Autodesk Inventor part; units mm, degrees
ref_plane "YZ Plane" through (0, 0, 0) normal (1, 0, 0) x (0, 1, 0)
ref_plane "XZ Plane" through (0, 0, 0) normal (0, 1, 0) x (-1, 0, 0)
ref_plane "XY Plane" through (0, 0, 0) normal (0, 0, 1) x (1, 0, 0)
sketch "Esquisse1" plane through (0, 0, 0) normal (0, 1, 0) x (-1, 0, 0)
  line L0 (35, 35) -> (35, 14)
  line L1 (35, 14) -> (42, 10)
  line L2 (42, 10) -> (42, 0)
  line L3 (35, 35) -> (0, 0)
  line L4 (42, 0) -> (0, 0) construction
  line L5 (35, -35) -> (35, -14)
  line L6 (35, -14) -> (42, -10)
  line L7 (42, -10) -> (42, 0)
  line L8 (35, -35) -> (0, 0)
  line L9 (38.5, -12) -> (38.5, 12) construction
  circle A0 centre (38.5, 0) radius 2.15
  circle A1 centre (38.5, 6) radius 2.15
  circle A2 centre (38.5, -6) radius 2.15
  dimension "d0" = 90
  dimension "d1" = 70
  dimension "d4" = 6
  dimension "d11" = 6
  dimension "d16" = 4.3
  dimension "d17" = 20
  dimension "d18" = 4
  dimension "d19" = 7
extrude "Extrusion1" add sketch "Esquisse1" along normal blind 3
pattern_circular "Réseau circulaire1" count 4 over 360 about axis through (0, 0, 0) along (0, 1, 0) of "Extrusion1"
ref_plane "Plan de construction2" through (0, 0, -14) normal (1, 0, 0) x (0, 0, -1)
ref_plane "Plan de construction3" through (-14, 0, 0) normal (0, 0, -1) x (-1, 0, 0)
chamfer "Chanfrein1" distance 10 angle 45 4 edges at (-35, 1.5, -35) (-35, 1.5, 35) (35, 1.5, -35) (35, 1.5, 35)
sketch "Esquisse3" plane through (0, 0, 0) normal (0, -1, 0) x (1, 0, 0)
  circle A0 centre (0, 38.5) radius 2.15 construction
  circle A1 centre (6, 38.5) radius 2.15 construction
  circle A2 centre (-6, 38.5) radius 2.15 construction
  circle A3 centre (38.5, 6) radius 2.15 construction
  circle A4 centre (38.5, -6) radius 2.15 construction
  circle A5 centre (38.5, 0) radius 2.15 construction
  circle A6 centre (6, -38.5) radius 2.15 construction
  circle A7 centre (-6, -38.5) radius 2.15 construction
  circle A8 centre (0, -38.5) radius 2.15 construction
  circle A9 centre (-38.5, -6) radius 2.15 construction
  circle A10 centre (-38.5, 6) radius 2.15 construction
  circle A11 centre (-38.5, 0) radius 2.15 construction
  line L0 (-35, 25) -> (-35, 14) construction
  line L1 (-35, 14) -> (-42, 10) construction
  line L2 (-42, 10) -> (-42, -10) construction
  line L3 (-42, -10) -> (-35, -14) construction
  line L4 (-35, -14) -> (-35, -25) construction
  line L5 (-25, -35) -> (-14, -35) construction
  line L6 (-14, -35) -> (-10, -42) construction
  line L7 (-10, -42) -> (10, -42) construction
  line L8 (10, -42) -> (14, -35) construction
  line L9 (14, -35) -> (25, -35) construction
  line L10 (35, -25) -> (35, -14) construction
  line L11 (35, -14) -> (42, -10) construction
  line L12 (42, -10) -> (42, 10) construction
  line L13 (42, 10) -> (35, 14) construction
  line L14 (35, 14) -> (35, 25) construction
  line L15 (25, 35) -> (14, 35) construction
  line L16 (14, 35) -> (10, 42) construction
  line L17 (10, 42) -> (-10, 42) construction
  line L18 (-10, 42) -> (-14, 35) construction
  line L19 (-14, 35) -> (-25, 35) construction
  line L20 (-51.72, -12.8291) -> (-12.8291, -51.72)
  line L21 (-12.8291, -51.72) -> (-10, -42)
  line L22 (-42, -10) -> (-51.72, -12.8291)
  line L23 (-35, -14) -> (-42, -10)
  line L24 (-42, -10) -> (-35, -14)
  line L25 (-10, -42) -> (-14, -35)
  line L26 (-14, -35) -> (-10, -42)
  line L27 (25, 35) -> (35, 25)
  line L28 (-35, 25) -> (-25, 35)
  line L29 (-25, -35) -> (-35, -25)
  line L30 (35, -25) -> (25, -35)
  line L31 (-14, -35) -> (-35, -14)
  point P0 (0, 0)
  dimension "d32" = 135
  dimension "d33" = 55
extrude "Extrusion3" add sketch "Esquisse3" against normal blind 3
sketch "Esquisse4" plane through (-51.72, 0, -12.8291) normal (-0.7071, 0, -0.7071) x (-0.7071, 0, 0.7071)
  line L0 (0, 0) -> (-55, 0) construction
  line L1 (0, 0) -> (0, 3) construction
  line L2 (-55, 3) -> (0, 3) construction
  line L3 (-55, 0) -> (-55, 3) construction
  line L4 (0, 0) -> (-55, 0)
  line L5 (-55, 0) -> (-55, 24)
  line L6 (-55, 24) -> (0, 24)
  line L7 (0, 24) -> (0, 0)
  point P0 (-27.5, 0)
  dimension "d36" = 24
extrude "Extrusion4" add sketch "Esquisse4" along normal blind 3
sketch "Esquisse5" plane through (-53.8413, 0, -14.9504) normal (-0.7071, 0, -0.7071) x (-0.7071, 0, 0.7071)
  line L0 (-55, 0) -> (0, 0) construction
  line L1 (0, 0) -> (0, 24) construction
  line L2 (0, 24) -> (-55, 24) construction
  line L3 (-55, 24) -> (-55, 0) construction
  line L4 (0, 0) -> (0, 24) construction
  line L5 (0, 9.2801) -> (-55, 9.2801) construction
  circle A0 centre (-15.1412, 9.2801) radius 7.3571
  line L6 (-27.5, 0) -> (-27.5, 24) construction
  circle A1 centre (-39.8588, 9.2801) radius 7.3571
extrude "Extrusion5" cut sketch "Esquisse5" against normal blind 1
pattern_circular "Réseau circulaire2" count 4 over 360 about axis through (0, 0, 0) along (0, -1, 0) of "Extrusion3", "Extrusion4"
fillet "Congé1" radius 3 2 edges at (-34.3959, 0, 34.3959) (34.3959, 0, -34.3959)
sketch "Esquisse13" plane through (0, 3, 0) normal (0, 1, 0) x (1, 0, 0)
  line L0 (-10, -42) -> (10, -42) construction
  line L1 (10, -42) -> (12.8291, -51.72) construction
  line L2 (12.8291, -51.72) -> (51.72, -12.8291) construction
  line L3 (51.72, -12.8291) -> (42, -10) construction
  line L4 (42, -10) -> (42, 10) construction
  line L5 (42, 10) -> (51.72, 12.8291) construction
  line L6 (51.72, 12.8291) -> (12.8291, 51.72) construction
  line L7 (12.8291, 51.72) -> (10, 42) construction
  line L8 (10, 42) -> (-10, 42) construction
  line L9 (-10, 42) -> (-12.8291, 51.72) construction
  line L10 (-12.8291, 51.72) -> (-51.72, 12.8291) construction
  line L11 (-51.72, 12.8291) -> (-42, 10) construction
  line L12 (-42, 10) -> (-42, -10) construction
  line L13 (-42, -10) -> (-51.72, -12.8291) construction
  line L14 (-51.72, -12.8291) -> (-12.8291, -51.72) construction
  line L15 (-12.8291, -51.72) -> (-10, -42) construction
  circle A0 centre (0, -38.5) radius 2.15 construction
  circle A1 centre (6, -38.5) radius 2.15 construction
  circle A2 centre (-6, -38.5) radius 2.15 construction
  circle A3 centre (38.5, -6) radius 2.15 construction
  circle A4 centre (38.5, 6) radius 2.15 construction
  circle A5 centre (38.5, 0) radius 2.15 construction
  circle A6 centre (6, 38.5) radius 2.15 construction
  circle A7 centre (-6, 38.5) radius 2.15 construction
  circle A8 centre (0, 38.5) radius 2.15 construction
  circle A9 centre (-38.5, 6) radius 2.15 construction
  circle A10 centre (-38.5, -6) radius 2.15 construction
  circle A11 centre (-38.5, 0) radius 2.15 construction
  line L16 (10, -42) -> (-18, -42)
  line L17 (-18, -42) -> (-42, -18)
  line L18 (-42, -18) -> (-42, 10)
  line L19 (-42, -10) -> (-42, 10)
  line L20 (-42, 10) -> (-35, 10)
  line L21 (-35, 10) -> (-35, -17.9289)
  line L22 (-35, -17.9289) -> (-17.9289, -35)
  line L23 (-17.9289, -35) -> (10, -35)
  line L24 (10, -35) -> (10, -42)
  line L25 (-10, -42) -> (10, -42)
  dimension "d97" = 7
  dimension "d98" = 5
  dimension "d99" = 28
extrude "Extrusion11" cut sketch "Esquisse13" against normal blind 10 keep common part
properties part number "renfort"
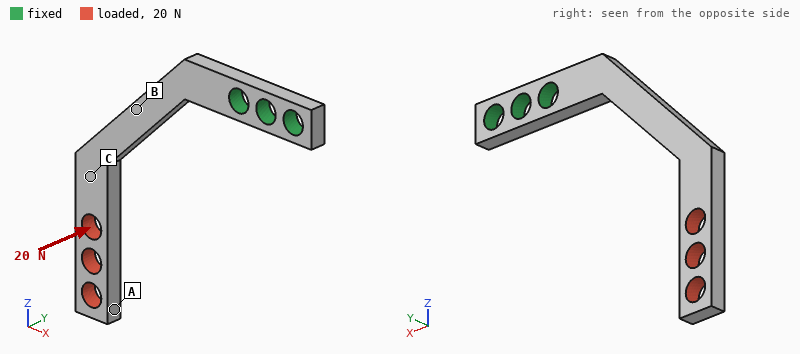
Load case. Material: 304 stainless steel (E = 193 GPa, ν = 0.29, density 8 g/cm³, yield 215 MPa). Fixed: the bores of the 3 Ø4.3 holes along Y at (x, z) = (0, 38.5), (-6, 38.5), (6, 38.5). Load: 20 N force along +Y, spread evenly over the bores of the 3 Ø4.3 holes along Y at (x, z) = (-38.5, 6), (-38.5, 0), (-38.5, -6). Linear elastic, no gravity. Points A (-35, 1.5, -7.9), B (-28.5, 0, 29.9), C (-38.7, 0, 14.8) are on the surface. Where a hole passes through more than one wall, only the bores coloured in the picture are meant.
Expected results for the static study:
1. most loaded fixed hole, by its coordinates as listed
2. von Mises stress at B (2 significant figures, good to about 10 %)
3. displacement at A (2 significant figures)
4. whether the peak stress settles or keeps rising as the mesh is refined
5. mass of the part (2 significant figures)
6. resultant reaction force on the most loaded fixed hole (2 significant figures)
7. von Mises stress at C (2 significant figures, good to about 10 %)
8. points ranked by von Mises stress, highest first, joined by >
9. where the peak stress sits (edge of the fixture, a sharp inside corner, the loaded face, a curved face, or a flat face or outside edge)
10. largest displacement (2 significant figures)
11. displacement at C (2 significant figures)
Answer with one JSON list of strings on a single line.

["(-6, 38.5)", "79 MPa", "0.47 mm", "keeps rising", "11 g", "22 N", "29 MPa", "B > C > A", "a sharp inside corner", "0.52 mm", "0.24 mm"]
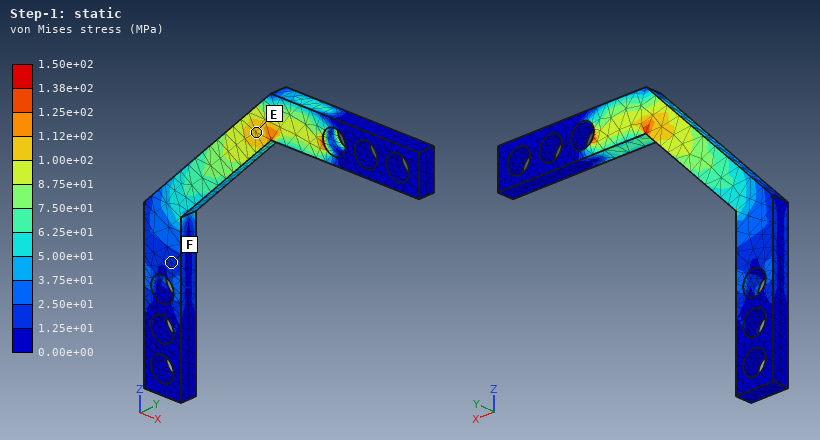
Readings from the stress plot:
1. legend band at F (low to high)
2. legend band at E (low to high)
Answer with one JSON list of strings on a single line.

["1.25e+01 to 2.50e+01 MPa", "1.00e+02 to 1.12e+02 MPa"]
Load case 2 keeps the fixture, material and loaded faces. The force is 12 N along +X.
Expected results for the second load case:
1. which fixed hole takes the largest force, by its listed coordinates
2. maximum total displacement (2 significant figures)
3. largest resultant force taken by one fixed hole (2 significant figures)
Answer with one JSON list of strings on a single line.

["(-6, 38.5)", "88 µm", "13 N"]
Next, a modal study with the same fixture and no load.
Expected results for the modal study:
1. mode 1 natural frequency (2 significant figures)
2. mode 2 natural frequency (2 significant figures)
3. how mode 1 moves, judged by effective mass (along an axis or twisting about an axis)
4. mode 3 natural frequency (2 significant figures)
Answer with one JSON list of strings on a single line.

["630 Hz", "1100 Hz", "along Y", "2600 Hz"]
